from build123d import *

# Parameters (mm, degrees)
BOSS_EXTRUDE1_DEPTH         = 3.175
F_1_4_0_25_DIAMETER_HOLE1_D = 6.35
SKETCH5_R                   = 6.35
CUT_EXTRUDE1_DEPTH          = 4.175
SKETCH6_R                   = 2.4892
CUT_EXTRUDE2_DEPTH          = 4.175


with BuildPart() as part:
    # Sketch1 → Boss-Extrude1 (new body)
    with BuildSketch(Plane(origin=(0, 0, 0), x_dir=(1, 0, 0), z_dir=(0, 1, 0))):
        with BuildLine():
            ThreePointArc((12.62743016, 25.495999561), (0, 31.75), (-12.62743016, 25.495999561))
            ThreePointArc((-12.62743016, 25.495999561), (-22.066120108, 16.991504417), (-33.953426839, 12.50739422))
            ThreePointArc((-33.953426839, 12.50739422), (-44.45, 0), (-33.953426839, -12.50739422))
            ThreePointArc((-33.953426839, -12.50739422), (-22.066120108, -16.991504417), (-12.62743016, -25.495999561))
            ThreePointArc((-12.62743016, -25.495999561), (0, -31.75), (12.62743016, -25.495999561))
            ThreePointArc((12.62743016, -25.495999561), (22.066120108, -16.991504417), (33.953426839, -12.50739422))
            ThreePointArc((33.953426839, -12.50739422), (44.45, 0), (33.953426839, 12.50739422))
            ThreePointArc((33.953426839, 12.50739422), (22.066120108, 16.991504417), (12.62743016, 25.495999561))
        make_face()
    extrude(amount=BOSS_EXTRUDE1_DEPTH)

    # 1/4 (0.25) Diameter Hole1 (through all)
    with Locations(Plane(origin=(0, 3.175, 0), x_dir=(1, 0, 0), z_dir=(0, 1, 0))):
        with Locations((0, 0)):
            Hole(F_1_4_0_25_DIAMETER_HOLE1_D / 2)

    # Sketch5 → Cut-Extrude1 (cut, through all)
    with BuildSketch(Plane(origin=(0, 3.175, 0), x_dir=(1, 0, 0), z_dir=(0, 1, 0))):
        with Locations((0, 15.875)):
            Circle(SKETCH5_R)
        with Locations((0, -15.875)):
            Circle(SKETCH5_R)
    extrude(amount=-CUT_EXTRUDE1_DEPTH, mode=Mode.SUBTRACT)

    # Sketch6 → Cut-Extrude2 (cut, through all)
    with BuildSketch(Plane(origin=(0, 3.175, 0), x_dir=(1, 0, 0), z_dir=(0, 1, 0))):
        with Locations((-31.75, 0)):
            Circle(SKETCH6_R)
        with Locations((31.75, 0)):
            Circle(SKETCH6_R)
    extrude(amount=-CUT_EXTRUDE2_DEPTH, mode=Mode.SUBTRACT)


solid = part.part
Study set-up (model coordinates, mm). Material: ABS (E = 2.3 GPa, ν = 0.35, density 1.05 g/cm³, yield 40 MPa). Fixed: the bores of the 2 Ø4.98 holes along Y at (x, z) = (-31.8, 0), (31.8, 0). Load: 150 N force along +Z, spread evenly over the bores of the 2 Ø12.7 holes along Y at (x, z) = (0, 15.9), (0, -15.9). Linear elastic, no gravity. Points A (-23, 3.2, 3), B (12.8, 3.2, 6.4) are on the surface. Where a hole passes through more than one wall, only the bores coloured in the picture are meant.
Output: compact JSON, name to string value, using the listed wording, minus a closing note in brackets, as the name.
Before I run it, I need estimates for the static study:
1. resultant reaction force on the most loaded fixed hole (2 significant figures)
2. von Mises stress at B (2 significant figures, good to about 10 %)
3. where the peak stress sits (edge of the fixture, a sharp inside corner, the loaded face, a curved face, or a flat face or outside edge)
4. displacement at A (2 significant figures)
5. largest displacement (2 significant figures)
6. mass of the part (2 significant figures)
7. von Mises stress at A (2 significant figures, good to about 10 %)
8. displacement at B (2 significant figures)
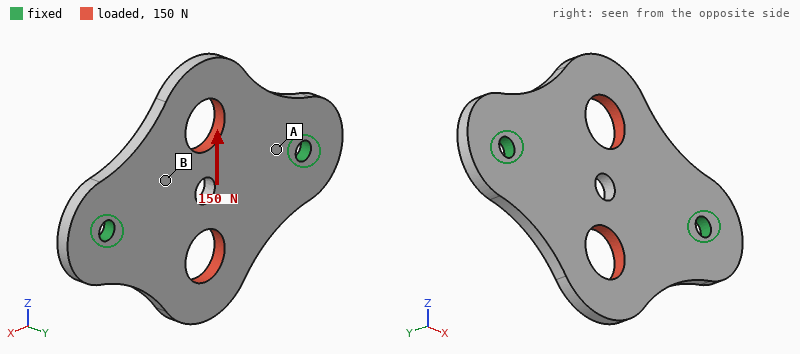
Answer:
{"resultant reaction force on the most loaded fixed hole": "75 N", "von Mises stress at B": "0.71 MPa", "where the peak stress sits": "edge of the fixture", "displacement at A": "15 µm", "largest displacement": "37 µm", "mass of the part": "10 g", "von Mises stress at A": "1.4 MPa", "displacement at B": "28 µm"}
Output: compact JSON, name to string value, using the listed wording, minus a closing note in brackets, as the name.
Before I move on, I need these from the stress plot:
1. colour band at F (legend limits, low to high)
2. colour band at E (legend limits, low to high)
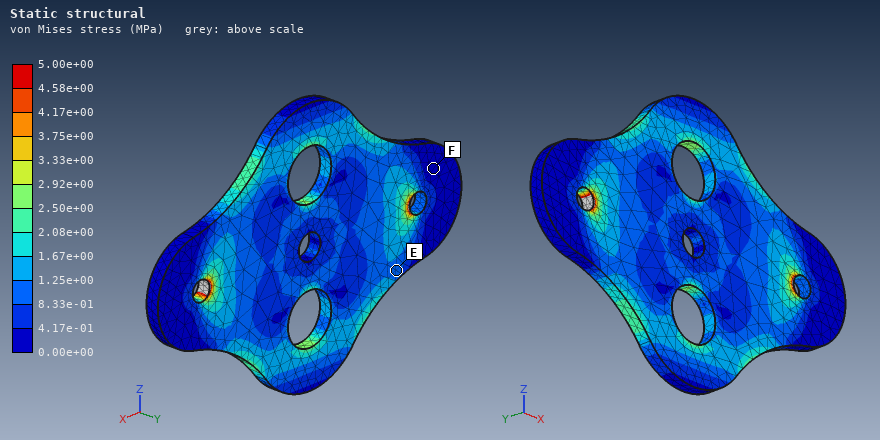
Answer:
{"colour band at F": "0.00e+00 to 4.17e-01 MPa", "colour band at E": "8.33e-01 to 1.25e+00 MPa"}
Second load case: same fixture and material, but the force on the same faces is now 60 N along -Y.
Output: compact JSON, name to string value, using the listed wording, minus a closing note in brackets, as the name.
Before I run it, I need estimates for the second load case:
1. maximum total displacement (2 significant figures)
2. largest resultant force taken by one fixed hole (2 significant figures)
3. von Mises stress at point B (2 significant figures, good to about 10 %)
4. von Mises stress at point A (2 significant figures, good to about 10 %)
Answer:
{"maximum total displacement": "0.67 mm", "largest resultant force taken by one fixed hole": "30 N", "von Mises stress at point B": "3.0 MPa", "von Mises stress at point A": "5.0 MPa"}
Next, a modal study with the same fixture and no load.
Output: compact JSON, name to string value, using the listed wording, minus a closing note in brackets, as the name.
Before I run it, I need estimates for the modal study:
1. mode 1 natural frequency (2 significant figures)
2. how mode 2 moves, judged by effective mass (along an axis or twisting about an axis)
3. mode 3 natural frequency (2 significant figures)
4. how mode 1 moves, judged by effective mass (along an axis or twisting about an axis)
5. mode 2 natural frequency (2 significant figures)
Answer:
{"mode 1 natural frequency": "680 Hz", "how mode 2 moves, judged by effective mass": "along Y", "mode 3 natural frequency": "1900 Hz", "how mode 1 moves, judged by effective mass": "twisting about X", "mode 2 natural frequency": "810 Hz"}
